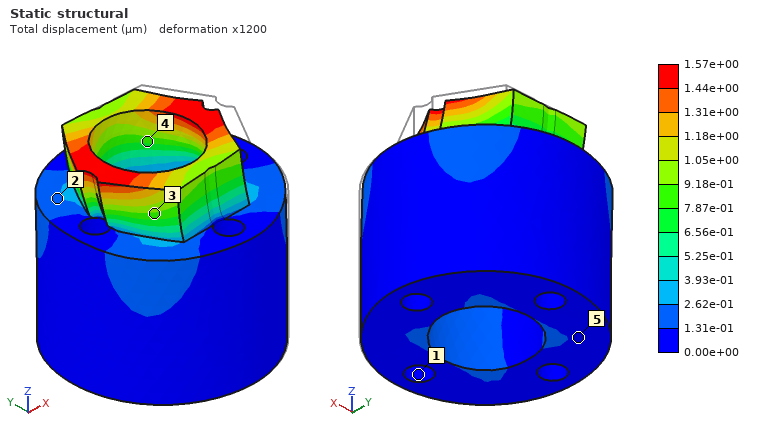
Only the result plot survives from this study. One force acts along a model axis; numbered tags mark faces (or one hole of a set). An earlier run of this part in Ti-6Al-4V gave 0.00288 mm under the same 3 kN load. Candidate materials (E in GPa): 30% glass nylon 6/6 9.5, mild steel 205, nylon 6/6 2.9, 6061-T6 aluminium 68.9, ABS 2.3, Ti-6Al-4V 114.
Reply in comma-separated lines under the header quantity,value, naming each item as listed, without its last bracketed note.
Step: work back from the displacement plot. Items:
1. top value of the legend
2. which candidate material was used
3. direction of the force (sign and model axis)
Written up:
quantity,value
top value of the legend,1.57e+00 µm
which candidate material was used,mild steel
direction of the force,-X
